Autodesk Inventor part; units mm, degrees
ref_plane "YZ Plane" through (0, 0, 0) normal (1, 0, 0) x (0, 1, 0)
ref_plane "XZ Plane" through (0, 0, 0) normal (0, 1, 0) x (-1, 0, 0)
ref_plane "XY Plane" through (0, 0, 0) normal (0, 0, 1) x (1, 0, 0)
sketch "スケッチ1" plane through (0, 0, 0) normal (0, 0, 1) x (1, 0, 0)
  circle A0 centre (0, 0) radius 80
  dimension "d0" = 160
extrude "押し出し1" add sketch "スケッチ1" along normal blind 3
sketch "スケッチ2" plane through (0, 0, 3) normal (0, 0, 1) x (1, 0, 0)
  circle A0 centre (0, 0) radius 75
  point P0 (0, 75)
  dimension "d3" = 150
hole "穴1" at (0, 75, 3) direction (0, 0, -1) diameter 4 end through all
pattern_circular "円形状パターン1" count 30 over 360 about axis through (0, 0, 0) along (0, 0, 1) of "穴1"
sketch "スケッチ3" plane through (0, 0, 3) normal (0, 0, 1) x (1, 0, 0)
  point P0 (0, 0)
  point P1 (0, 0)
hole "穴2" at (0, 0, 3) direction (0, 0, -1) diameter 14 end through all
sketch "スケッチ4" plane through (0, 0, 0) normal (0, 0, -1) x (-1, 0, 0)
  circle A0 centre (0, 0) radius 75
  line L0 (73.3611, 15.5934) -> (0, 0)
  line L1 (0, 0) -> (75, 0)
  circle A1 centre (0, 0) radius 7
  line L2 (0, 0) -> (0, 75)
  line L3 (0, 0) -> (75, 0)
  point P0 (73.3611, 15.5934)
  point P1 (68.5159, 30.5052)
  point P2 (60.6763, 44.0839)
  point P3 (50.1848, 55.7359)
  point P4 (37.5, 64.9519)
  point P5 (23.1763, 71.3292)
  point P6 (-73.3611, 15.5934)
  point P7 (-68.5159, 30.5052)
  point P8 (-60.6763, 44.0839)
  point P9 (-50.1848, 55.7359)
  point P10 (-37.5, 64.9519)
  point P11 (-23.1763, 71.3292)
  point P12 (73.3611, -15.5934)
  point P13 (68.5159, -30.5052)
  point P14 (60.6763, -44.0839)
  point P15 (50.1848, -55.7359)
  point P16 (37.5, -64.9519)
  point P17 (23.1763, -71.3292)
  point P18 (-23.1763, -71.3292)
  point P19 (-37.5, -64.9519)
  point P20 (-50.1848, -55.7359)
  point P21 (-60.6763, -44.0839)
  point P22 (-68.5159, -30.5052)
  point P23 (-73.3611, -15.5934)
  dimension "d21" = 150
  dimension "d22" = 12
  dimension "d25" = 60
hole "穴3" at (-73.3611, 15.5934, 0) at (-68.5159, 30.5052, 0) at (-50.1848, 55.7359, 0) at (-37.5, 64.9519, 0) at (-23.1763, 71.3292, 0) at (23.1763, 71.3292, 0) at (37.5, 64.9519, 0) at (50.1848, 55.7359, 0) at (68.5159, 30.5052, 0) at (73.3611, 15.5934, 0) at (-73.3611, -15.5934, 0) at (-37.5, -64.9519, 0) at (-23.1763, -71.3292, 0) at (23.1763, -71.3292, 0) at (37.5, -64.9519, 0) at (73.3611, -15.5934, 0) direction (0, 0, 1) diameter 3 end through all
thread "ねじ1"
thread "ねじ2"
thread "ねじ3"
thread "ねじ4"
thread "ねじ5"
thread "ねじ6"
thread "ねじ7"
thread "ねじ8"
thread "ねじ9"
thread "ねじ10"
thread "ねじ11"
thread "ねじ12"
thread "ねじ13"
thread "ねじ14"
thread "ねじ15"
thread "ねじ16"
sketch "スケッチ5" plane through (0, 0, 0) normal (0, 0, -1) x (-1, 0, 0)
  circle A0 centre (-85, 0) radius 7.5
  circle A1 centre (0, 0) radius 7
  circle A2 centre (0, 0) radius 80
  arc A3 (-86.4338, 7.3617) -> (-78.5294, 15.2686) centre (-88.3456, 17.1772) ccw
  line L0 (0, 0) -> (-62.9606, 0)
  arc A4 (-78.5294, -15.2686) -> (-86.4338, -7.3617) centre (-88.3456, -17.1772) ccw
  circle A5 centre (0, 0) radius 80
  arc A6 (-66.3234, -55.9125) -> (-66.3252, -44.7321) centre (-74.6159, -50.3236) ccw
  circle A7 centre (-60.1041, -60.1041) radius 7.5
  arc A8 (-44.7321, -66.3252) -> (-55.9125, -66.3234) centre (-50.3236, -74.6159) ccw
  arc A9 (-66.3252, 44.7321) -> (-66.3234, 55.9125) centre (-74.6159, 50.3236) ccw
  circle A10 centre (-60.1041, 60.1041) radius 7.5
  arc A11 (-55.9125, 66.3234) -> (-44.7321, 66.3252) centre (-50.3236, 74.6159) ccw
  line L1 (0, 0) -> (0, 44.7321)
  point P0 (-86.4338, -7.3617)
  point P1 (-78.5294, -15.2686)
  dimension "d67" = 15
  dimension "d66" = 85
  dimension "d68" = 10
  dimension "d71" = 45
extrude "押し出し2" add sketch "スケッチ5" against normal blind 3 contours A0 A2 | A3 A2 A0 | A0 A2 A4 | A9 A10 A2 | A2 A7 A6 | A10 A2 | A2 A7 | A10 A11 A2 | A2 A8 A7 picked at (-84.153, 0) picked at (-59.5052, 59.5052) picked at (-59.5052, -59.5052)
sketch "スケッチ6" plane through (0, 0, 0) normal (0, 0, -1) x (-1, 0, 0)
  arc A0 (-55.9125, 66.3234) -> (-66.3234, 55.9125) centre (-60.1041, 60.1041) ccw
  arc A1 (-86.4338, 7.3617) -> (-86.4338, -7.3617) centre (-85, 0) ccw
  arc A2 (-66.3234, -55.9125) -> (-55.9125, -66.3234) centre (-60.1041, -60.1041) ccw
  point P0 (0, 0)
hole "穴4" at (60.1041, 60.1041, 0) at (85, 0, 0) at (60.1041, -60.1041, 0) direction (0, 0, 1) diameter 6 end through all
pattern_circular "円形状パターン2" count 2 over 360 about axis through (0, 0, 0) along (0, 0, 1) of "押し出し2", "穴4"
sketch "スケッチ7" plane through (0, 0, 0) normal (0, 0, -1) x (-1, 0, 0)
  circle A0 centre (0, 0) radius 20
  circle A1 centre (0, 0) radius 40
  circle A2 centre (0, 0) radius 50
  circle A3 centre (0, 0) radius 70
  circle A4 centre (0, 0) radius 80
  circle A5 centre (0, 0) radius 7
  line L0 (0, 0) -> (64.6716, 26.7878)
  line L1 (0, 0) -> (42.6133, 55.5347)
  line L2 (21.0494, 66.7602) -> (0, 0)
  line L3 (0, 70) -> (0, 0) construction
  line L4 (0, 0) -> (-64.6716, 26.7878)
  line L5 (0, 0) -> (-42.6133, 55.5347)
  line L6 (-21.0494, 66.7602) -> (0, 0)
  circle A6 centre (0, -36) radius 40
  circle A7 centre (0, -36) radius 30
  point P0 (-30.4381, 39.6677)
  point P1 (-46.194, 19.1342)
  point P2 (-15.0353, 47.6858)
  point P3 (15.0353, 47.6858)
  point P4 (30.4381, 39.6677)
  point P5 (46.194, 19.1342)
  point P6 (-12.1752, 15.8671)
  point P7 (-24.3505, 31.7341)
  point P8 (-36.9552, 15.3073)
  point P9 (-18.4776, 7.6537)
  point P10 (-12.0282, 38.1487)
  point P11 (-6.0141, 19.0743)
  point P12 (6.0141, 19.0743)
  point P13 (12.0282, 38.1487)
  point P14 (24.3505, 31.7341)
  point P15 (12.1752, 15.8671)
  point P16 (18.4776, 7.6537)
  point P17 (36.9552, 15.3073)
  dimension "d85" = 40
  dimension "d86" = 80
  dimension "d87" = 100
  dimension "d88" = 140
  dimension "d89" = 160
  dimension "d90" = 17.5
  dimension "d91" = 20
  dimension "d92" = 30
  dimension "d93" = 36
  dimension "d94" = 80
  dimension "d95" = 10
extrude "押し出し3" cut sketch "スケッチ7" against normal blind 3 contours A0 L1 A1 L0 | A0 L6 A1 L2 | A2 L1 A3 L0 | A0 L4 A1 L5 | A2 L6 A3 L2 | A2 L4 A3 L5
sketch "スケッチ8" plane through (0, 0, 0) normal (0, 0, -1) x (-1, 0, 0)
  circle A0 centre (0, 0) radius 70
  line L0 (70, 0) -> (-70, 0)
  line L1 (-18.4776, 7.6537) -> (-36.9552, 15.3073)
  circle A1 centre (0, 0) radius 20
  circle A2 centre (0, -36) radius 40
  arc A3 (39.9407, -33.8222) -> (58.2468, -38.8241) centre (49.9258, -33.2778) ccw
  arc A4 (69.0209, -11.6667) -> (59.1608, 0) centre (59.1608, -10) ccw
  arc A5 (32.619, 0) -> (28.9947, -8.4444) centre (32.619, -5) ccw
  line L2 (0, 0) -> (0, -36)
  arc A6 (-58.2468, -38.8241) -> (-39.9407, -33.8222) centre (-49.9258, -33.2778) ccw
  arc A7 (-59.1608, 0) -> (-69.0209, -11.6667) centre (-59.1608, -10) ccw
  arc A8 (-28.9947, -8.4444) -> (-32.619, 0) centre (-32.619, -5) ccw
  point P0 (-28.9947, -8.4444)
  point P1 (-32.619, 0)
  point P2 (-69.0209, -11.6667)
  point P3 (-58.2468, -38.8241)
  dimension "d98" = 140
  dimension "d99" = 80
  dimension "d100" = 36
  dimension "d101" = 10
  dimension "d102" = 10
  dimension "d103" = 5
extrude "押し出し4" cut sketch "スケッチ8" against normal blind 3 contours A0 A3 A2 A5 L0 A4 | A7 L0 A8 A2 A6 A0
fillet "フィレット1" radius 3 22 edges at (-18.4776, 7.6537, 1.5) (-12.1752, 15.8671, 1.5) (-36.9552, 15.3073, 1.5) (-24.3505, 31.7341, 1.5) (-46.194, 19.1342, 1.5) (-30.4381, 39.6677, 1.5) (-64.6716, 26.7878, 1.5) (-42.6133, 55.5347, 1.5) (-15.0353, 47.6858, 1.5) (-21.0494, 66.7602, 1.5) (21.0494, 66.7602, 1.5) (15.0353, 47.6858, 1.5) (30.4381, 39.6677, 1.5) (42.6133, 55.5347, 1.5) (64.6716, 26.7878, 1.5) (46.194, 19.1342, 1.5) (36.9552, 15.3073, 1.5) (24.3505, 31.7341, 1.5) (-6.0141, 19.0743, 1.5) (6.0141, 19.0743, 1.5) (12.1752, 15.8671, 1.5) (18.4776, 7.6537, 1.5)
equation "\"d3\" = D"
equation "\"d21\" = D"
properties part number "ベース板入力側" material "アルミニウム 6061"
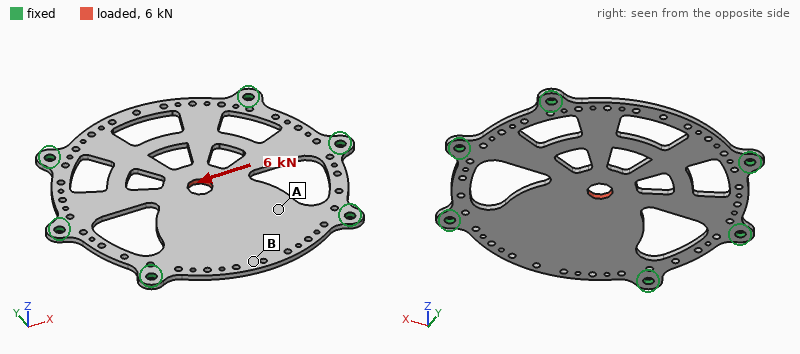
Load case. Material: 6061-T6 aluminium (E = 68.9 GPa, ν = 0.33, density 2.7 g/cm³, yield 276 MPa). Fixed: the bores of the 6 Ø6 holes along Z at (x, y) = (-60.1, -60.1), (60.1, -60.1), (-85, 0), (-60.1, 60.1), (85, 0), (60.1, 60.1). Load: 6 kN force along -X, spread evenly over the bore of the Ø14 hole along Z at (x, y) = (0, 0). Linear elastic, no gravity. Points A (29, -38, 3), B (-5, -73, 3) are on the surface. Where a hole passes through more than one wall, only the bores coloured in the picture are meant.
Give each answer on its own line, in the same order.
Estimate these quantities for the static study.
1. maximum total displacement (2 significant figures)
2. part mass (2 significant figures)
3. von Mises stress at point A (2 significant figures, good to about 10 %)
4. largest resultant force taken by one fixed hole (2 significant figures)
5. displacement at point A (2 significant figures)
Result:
48 µm
120 g
21 MPa
1.4 kN
17 µm
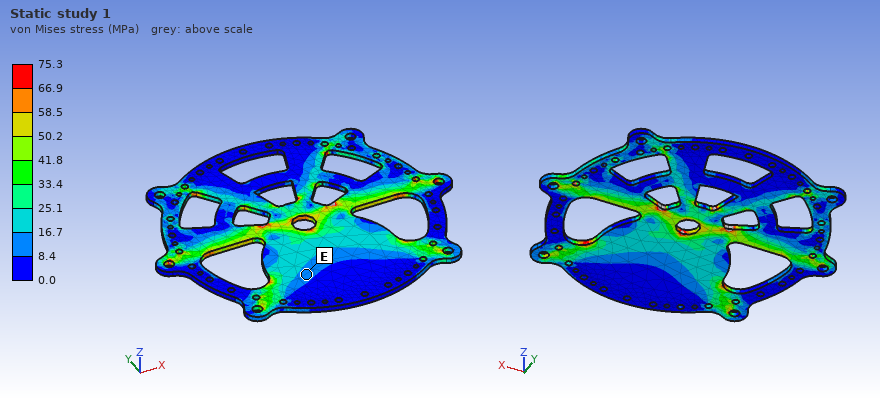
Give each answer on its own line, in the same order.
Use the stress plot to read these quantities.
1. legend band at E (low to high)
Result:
8.4 to 16.7 MPa
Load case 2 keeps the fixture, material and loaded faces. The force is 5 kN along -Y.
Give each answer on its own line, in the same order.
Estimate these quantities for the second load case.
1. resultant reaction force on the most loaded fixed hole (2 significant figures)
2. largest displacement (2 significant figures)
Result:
1.7 kN
56 µm
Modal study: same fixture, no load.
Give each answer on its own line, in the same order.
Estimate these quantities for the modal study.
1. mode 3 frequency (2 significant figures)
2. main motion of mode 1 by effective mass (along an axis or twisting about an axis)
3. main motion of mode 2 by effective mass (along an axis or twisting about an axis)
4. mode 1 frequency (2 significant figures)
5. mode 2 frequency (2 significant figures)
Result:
1200 Hz
along Z
twisting about X
680 Hz
1000 Hz
